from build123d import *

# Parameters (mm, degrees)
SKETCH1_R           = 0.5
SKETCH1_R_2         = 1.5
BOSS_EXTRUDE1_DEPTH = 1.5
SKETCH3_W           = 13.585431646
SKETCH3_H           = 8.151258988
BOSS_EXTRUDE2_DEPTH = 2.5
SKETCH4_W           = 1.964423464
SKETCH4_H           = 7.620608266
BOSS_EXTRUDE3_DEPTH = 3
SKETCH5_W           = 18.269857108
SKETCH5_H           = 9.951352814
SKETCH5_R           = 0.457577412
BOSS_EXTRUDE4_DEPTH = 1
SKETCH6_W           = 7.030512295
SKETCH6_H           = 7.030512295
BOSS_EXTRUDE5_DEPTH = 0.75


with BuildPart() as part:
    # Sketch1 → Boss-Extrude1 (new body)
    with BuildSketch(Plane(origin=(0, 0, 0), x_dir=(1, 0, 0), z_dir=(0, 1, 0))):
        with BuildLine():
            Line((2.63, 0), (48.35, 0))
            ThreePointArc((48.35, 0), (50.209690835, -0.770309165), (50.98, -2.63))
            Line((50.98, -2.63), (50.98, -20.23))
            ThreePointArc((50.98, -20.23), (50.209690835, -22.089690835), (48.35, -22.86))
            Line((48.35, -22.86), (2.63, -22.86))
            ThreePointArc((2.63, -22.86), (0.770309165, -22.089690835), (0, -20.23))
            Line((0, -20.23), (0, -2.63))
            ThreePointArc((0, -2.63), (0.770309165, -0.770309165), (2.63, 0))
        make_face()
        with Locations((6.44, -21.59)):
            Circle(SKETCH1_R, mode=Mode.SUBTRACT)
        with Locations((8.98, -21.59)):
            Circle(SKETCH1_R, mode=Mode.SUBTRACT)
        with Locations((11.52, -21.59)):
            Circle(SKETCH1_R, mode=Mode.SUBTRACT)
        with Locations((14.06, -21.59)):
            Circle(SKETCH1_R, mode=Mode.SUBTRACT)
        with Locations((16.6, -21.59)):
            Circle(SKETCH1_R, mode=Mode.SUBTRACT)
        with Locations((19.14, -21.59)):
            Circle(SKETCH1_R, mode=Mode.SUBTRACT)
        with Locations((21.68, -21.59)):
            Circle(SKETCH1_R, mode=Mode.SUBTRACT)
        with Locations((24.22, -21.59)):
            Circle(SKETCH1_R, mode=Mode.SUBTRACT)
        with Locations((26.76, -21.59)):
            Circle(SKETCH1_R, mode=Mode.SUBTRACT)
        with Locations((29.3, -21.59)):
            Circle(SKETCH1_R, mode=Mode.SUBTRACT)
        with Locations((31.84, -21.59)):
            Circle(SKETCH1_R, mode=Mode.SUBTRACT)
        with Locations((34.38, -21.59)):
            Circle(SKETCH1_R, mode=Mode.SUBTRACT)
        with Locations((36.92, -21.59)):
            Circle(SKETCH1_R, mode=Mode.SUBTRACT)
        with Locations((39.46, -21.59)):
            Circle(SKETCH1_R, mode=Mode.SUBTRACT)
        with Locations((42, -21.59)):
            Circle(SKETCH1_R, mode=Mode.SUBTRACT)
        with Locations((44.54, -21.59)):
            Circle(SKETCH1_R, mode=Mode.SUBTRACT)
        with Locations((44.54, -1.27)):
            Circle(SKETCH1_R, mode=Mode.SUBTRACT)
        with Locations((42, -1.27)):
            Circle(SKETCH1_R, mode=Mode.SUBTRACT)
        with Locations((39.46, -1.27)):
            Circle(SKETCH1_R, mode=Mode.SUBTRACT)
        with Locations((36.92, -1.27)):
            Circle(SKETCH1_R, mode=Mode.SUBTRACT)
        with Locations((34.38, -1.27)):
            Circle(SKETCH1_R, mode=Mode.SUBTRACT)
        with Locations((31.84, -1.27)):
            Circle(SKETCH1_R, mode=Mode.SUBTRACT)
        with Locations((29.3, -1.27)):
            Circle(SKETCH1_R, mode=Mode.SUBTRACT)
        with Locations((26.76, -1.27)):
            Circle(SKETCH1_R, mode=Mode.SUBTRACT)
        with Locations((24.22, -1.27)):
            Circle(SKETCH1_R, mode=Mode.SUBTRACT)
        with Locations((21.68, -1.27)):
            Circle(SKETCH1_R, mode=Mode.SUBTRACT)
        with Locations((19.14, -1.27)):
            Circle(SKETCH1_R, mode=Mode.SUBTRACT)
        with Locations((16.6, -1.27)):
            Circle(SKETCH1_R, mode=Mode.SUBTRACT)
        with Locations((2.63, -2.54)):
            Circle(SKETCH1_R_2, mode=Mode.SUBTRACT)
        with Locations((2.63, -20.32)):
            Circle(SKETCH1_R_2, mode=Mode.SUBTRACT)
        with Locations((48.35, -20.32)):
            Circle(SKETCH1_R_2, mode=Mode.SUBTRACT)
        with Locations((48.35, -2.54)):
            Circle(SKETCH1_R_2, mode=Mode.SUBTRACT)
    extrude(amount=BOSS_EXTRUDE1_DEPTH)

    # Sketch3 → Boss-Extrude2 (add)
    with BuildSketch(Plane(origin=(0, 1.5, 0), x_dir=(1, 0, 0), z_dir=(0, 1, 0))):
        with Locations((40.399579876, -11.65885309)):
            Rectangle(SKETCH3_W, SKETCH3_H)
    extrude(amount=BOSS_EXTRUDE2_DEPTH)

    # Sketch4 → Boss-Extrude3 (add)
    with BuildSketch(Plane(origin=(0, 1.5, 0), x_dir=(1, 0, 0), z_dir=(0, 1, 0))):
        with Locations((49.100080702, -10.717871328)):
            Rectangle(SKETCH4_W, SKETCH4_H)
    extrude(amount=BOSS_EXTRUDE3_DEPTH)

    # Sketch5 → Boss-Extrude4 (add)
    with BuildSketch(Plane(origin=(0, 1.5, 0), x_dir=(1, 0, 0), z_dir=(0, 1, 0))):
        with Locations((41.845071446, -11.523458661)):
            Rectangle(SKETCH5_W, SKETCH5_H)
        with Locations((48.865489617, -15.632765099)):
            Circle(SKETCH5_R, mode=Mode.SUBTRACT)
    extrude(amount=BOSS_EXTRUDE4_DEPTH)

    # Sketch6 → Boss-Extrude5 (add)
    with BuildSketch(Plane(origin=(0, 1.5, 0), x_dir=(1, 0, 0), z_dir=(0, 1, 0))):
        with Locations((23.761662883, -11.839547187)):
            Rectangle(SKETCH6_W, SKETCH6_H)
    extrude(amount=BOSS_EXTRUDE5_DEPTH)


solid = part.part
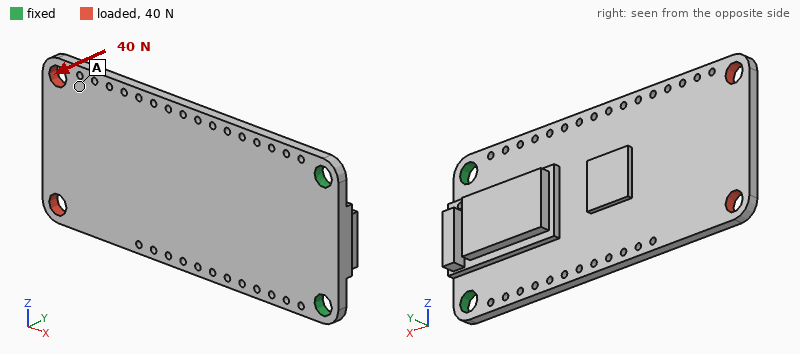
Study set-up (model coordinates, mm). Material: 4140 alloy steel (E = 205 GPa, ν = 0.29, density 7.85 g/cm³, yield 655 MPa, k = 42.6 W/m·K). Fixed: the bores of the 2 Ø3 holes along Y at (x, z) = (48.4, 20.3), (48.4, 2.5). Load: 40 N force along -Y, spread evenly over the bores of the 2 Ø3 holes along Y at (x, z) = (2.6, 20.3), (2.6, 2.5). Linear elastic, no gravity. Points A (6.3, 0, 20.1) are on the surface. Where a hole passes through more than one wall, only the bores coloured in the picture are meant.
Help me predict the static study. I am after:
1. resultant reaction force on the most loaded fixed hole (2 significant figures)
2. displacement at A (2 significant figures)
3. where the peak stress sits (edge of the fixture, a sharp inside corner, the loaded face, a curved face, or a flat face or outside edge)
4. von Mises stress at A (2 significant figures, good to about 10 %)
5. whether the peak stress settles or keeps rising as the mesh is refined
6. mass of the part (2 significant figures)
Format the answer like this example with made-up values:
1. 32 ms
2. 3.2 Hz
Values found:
1. 25 N
2. 0.43 mm
3. edge of the fixture
4. 22 MPa
5. keeps rising
6. 16 g
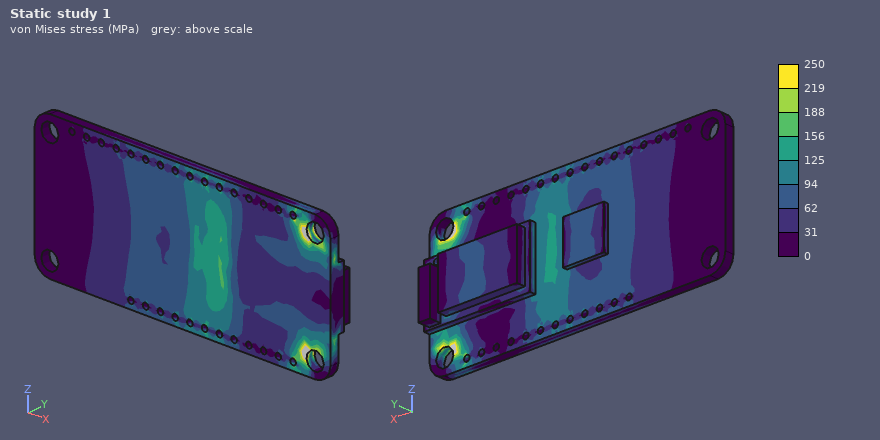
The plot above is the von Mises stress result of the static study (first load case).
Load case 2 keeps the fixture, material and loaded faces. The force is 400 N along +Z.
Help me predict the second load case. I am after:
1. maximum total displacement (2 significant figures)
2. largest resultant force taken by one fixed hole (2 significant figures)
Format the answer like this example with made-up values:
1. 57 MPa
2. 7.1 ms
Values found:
1. 59 µm
2. 1.0 kN
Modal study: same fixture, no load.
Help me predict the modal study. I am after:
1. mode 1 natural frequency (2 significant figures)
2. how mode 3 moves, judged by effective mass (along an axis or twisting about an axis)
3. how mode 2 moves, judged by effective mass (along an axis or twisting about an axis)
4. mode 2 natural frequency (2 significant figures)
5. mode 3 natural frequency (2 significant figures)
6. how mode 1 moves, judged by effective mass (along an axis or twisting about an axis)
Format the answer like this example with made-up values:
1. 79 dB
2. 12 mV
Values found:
1. 790 Hz
2. along Y
3. twisting about X
4. 3400 Hz
5. 3600 Hz
6. along Y
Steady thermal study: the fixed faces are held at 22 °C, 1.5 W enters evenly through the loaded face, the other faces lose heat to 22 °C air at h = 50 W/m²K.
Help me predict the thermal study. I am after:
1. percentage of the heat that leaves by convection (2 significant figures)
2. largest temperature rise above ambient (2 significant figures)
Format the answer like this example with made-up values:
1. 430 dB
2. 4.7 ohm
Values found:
1. 73 %
2. 27 K
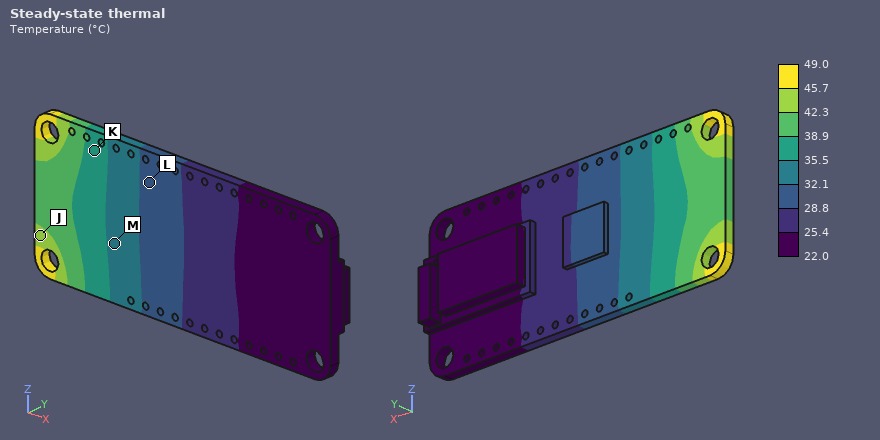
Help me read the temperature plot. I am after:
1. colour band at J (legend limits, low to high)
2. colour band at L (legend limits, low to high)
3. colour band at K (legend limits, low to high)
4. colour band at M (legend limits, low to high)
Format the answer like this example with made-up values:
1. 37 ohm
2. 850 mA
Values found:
1. 42.3 to 45.7 °C
2. 28.8 to 32.1 °C
3. 35.5 to 38.9 °C
4. 32.1 to 35.5 °C
